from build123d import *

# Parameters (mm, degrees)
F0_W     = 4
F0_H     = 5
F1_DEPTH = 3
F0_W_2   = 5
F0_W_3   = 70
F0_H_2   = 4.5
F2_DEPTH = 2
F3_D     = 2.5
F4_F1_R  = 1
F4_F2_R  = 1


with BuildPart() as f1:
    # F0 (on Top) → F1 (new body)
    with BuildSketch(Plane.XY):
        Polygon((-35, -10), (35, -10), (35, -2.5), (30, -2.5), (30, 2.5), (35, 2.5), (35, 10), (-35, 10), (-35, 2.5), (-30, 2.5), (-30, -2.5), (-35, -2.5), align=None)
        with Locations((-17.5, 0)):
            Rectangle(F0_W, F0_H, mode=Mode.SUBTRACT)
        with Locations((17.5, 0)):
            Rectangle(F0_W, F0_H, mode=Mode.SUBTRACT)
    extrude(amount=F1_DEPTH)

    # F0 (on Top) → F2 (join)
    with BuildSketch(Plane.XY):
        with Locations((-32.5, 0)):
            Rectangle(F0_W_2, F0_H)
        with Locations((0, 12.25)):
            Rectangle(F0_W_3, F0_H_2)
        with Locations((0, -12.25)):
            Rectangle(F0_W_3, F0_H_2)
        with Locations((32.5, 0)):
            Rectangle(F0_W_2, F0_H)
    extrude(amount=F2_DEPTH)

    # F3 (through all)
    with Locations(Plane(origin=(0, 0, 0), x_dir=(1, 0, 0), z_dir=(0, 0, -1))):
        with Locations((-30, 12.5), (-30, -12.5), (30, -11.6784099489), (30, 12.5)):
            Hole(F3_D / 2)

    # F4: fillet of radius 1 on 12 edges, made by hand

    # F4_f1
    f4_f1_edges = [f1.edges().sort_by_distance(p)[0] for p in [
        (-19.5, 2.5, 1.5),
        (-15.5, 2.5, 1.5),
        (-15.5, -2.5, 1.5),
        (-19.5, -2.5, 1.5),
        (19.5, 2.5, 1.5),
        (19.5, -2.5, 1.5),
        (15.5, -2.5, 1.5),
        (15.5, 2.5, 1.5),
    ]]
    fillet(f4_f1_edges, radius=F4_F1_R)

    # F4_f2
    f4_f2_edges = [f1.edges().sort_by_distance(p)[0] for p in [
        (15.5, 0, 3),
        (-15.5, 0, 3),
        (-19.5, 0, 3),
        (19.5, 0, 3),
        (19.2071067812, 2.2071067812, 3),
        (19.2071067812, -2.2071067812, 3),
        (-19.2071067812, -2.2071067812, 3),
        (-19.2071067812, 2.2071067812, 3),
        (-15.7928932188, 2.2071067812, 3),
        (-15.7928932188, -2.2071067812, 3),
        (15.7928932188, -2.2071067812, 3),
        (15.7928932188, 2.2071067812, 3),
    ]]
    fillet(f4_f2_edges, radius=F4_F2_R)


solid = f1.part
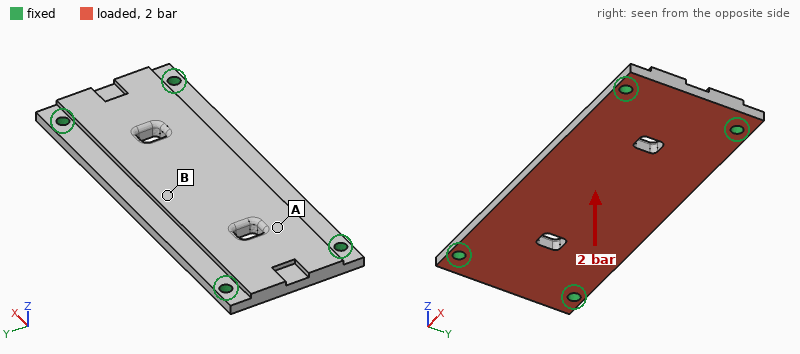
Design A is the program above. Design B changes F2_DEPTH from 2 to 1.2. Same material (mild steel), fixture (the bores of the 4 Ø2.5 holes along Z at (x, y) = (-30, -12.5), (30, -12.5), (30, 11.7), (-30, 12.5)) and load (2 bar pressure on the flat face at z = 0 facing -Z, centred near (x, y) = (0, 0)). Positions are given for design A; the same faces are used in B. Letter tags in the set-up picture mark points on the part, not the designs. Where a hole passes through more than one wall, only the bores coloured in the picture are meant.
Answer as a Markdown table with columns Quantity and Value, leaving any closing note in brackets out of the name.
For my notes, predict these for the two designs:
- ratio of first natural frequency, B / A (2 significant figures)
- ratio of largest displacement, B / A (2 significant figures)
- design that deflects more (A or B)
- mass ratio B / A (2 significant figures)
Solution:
| Quantity | Value |
|---|---|
| ratio of first natural frequency, B / A | 0.88 |
| ratio of largest displacement, B / A | 1.4 |
| design that deflects more | B |
| mass ratio B / A | 0.90 |
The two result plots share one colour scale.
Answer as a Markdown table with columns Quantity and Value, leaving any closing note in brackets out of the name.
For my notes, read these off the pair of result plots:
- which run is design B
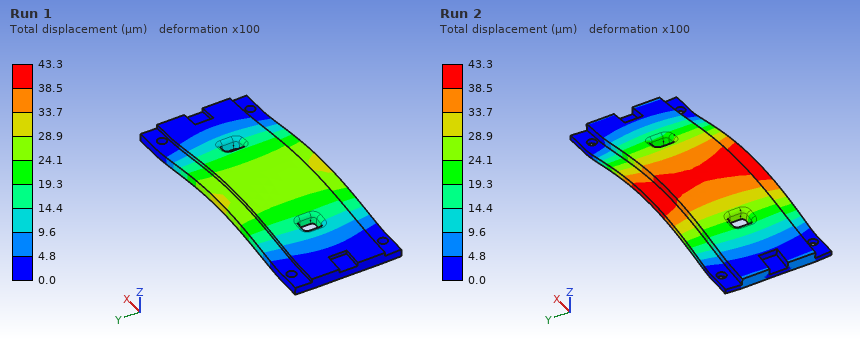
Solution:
| Quantity | Value |
|---|---|
| which run is design B | Run 2 |
